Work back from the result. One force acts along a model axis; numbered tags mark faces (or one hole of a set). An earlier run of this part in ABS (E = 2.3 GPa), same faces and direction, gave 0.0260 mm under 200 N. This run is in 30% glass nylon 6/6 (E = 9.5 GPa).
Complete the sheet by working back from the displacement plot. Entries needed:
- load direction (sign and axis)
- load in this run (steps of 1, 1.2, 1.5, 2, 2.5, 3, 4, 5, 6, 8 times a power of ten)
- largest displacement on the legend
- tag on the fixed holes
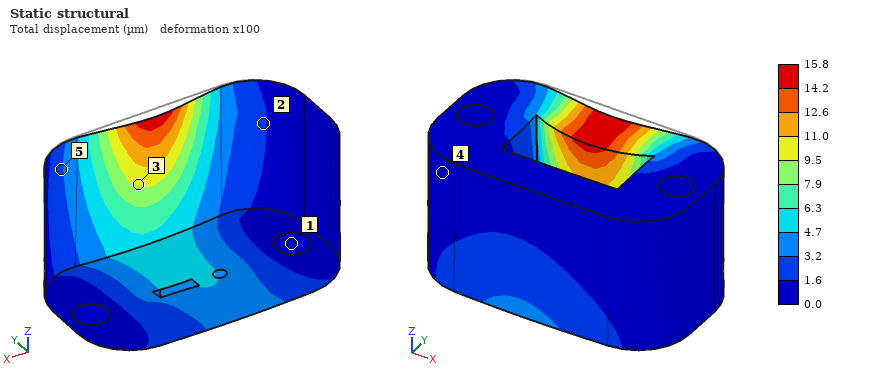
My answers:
-Y
500 N
15.8 µm
1
